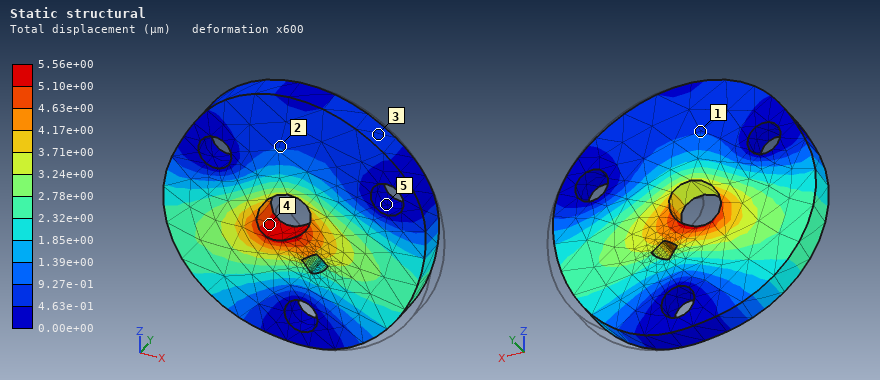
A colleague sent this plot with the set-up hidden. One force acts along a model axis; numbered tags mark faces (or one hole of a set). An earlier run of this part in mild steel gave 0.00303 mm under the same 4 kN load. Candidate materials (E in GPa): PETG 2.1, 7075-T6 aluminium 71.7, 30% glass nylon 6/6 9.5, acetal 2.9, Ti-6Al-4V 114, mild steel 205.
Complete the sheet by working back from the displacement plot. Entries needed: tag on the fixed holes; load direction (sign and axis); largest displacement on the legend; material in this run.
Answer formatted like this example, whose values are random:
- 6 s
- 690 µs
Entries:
- 5
- -X
- 5.56e+00 µm
- Ti-6Al-4V
